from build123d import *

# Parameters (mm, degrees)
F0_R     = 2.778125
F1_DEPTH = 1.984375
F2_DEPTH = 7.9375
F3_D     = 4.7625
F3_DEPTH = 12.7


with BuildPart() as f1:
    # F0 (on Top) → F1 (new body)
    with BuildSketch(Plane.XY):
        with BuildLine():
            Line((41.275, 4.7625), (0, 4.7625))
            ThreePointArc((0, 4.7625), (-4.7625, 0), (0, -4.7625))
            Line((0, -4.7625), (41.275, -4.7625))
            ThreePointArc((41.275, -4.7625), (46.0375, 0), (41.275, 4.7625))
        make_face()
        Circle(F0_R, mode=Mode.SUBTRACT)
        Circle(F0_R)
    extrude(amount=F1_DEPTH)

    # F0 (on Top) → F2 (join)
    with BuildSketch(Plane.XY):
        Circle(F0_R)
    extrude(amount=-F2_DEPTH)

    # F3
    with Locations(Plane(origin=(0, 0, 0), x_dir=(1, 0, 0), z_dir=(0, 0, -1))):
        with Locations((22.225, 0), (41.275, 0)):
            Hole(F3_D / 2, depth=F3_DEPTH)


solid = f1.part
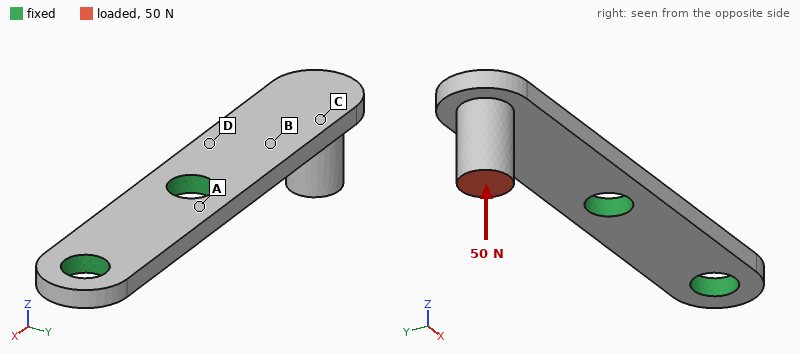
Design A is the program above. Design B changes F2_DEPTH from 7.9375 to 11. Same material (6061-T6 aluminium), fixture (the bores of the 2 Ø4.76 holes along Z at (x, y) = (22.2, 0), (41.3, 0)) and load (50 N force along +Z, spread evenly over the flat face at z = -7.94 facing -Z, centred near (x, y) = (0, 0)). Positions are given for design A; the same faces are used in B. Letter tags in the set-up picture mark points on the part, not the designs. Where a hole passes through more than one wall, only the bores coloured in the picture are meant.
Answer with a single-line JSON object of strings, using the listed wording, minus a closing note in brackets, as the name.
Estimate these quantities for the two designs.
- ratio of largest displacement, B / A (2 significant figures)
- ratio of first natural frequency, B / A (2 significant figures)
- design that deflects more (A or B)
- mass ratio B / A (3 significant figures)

{"ratio of largest displacement, B / A": "1.1", "ratio of first natural frequency, B / A": "0.88", "design that deflects more": "B", "mass ratio B / A": "1.07"}
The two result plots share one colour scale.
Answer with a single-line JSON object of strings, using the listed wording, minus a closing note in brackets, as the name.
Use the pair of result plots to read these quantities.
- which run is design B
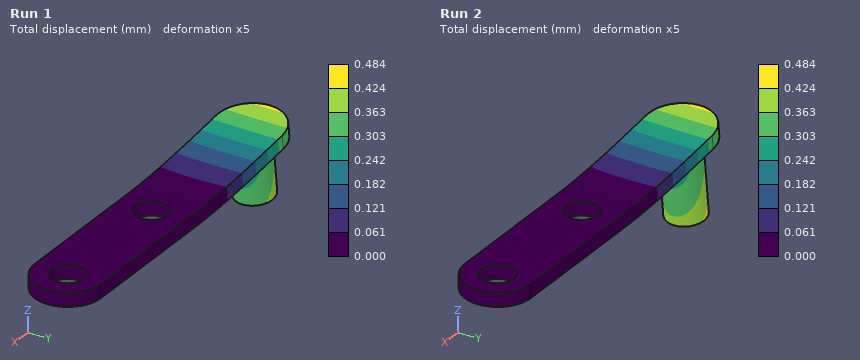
{"which run is design B": "Run 2"}
